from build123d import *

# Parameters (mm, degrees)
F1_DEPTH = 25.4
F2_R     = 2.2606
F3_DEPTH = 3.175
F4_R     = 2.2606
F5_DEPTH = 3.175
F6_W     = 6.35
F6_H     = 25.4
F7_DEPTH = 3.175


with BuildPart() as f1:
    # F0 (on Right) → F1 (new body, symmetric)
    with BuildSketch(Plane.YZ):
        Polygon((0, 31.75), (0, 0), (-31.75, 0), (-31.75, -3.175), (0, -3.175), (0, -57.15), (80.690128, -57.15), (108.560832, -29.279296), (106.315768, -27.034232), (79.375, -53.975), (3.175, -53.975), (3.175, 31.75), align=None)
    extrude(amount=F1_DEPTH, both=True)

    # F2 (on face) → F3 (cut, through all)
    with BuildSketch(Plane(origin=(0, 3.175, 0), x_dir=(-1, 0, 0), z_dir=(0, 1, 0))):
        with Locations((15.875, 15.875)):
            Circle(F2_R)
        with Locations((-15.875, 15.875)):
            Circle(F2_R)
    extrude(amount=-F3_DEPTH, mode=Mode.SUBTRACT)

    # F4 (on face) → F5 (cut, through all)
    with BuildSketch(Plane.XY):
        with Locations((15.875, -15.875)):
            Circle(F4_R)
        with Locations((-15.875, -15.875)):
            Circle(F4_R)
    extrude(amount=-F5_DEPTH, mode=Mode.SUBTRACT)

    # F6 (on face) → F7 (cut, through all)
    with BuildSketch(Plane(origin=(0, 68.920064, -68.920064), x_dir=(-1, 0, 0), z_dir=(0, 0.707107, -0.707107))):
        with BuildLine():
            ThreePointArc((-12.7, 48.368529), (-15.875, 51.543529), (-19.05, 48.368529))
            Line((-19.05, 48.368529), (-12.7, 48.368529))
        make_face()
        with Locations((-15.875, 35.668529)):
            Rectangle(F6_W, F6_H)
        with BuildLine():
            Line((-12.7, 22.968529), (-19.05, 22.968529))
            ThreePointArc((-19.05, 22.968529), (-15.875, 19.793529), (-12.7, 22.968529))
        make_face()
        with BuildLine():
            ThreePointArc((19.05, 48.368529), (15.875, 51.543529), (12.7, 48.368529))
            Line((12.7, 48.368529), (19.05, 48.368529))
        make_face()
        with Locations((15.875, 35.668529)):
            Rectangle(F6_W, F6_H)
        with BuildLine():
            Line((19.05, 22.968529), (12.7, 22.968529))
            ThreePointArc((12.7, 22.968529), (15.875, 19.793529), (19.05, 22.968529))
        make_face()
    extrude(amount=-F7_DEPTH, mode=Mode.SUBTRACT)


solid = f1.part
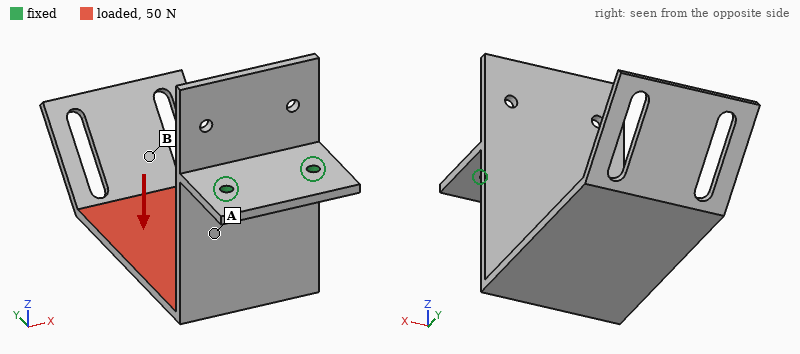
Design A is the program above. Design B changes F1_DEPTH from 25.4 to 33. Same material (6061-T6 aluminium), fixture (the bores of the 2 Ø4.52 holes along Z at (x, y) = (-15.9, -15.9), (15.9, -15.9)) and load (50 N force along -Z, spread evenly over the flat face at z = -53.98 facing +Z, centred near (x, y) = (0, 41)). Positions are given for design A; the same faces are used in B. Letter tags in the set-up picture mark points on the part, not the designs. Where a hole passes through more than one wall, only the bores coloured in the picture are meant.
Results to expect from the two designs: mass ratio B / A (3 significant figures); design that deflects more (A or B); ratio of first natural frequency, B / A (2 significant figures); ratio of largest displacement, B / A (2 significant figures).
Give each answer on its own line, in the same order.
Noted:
1.31
A
0.98
0.77
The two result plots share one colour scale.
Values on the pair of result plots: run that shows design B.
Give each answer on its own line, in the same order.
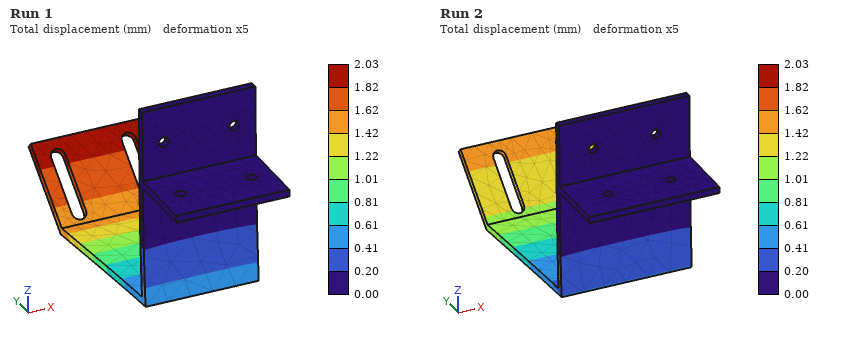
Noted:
Run 2
